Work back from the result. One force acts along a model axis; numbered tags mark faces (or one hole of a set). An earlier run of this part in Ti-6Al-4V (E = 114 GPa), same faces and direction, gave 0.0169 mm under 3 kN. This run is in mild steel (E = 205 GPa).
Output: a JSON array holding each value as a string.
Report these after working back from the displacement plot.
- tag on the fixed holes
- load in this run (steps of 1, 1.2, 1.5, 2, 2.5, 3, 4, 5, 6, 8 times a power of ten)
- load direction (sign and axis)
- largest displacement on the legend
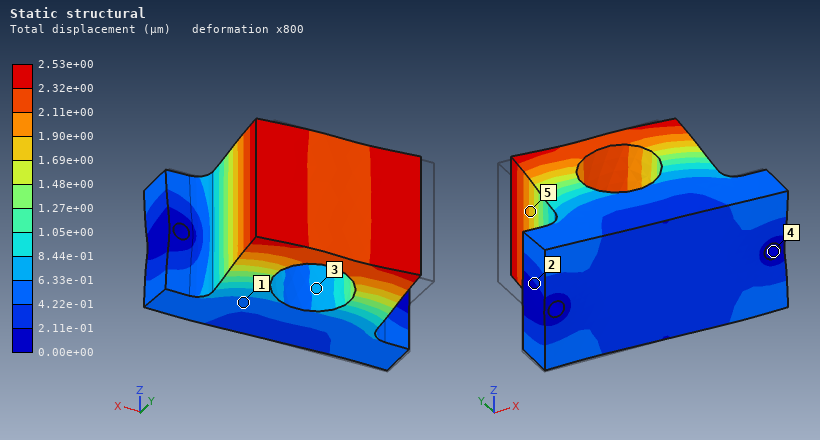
["4", "800 N", "+X", "2.53e+00 µm"]
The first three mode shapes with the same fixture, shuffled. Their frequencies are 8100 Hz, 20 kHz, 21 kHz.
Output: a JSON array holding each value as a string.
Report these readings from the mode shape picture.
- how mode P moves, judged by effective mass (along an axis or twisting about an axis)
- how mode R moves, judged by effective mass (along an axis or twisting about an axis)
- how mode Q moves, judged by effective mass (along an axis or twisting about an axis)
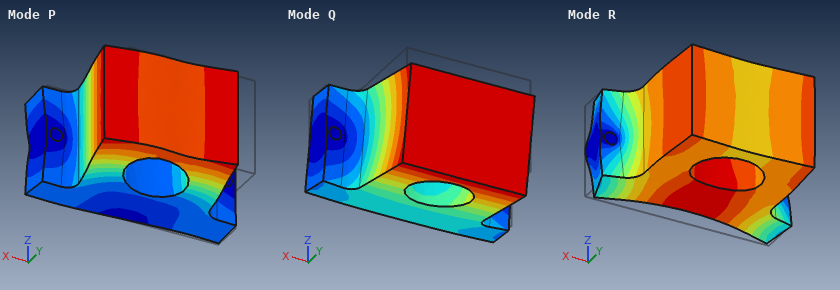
["along X", "along Y", "along Z"]
